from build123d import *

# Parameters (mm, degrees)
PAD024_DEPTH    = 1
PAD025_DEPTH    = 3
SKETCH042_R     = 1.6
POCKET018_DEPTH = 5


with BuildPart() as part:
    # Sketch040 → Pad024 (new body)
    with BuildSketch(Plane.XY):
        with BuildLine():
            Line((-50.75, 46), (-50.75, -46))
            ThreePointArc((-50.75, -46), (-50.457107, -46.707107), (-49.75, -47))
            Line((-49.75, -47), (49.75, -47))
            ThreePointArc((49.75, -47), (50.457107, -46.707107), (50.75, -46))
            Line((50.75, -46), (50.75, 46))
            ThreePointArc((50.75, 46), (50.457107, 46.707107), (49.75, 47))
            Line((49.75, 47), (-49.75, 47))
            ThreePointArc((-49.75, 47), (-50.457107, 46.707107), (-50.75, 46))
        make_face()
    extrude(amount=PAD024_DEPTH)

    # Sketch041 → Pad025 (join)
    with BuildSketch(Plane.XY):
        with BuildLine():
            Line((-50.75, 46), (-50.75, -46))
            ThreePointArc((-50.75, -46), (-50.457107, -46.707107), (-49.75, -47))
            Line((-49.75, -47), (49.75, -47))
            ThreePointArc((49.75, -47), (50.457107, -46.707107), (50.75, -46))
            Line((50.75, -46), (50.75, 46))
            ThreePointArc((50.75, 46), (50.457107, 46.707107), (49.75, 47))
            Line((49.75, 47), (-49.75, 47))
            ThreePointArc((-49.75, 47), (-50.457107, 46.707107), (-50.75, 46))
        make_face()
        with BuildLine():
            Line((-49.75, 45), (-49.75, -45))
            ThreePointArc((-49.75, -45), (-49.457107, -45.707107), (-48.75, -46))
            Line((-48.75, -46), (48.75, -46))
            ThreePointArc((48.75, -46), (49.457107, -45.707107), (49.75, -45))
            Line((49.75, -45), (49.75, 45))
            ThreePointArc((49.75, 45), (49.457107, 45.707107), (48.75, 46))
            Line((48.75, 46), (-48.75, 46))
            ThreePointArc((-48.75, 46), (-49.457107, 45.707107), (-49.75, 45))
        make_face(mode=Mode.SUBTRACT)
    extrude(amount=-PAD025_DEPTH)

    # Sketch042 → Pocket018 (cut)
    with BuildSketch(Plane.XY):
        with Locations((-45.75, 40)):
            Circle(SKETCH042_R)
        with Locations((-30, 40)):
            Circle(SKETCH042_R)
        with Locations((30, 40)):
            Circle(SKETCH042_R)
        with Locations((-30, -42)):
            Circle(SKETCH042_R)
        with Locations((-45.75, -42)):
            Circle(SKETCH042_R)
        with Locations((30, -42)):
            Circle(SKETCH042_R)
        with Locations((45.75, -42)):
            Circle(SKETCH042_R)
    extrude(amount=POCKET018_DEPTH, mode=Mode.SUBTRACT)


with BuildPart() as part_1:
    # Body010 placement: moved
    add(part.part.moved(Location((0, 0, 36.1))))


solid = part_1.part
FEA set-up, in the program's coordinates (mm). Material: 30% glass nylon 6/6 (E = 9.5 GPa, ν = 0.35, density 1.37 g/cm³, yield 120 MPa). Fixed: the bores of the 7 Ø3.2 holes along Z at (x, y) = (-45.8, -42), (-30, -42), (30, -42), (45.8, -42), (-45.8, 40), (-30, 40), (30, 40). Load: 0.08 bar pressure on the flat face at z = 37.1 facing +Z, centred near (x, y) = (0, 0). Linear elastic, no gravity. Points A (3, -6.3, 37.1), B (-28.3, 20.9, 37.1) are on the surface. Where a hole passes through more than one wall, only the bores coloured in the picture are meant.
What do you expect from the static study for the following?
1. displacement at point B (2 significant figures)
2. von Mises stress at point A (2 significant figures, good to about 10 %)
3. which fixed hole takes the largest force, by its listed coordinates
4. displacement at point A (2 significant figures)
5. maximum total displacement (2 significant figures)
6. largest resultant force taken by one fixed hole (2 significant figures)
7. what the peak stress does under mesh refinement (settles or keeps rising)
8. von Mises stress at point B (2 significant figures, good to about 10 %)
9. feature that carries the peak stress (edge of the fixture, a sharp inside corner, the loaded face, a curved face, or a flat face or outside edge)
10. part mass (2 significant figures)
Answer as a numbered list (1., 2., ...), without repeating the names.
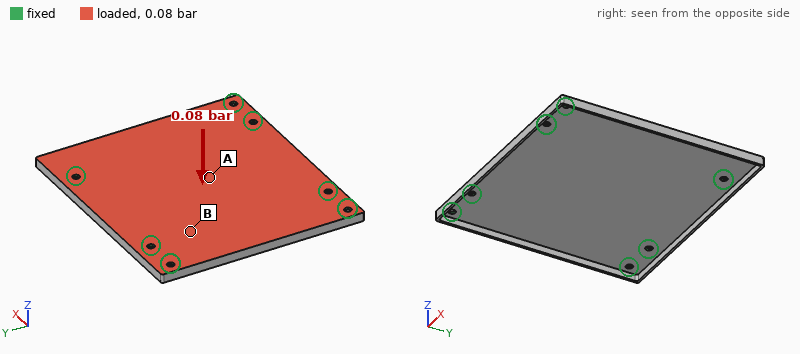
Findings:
1. 0.58 mm
2. 13 MPa
3. (30, 40)
4. 1.5 mm
5. 1.5 mm
6. 21 N
7. keeps rising
8. 5.8 MPa
9. edge of the fixture
10. 15 g
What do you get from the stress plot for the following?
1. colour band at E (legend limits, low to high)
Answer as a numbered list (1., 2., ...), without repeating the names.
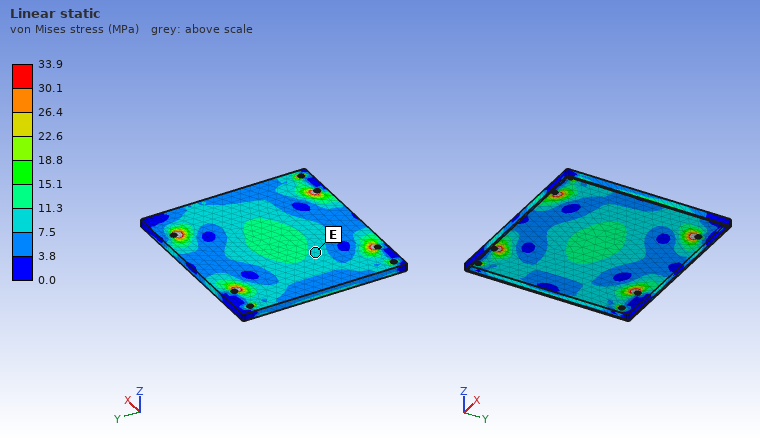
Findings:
1. 7.5 to 11.3 MPa
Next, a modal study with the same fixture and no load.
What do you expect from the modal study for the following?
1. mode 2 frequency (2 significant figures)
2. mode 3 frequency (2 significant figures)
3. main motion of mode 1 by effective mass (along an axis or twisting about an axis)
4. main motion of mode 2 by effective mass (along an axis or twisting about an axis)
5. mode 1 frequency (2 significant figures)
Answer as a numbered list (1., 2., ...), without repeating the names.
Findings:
1. 640 Hz
2. 820 Hz
3. along Z
4. twisting about Y
5. 390 Hz
